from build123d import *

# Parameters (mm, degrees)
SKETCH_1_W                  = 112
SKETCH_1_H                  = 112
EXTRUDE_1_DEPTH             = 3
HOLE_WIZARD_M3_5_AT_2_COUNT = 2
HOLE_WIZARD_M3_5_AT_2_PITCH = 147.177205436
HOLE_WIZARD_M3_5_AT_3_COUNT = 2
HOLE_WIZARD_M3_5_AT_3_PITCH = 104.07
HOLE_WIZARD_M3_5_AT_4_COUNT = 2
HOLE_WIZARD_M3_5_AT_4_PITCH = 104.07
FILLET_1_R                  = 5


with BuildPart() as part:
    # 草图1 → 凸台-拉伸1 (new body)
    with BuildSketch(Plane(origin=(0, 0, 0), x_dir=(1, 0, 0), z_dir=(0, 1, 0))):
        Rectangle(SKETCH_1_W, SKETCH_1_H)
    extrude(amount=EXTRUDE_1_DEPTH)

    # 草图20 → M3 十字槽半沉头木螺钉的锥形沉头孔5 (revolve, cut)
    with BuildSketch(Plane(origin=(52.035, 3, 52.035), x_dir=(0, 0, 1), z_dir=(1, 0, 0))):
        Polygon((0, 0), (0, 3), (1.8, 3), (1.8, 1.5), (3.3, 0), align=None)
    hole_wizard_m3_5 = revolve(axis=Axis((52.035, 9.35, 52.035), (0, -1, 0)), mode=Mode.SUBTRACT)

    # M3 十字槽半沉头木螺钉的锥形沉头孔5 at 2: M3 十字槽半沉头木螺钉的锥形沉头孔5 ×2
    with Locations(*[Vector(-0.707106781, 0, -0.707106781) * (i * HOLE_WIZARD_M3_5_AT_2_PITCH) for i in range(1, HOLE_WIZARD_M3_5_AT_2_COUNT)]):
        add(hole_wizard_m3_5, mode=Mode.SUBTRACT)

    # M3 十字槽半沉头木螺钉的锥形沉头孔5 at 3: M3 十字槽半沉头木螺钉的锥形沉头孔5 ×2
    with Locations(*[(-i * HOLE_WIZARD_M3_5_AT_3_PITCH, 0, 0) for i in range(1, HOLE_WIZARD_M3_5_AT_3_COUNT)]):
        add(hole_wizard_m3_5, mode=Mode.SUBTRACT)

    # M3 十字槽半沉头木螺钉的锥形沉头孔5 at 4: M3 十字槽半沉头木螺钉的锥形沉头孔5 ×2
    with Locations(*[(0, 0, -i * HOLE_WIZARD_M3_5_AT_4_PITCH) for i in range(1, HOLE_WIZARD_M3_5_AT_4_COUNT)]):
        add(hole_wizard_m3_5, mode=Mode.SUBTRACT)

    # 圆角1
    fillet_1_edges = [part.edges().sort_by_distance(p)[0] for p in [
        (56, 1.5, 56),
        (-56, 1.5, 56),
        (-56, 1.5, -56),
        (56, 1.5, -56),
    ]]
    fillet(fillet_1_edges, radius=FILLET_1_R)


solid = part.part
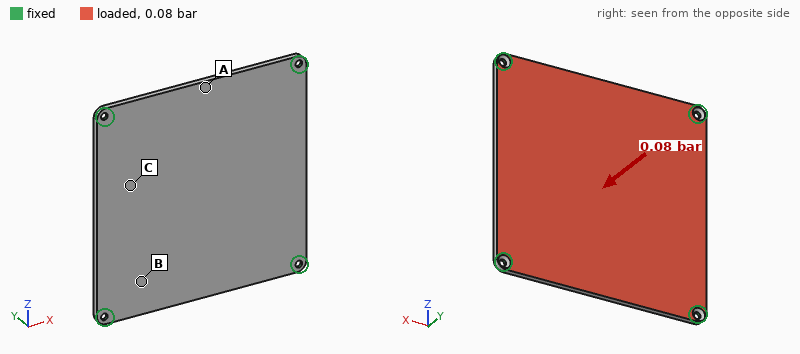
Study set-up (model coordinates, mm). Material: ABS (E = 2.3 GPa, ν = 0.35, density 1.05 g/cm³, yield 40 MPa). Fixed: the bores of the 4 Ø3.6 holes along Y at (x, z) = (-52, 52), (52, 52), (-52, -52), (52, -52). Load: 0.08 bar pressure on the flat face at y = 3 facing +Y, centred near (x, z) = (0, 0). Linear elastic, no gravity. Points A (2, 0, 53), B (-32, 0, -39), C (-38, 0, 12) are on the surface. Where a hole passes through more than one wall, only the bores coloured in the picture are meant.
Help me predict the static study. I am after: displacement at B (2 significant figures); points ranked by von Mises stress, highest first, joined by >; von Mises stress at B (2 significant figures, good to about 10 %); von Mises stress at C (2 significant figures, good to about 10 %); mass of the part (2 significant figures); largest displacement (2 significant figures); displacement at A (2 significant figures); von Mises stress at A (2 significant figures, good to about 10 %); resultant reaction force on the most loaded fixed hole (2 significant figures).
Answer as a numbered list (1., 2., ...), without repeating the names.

1. 0.79 mm
2. A > C > B
3. 1.4 MPa
4. 3.3 MPa
5. 39 g
6. 1.8 mm
7. 1.0 mm
8. 4.4 MPa
9. 49 N
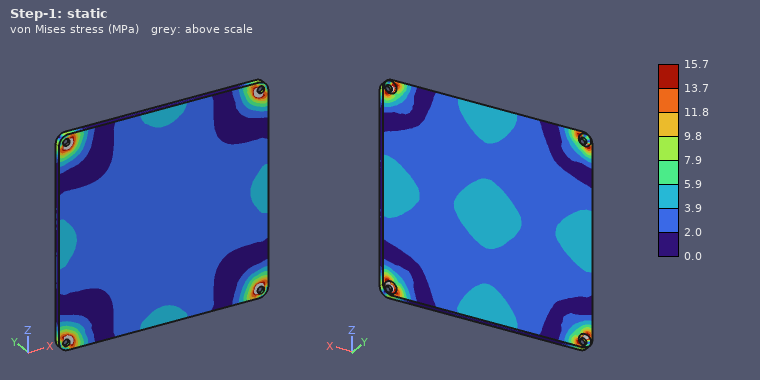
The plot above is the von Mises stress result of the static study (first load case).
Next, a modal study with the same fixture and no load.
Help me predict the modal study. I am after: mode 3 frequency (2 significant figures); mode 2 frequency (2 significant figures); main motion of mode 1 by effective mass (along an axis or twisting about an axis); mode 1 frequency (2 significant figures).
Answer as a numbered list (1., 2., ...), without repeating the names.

1. 420 Hz
2. 420 Hz
3. along Y
4. 230 Hz
